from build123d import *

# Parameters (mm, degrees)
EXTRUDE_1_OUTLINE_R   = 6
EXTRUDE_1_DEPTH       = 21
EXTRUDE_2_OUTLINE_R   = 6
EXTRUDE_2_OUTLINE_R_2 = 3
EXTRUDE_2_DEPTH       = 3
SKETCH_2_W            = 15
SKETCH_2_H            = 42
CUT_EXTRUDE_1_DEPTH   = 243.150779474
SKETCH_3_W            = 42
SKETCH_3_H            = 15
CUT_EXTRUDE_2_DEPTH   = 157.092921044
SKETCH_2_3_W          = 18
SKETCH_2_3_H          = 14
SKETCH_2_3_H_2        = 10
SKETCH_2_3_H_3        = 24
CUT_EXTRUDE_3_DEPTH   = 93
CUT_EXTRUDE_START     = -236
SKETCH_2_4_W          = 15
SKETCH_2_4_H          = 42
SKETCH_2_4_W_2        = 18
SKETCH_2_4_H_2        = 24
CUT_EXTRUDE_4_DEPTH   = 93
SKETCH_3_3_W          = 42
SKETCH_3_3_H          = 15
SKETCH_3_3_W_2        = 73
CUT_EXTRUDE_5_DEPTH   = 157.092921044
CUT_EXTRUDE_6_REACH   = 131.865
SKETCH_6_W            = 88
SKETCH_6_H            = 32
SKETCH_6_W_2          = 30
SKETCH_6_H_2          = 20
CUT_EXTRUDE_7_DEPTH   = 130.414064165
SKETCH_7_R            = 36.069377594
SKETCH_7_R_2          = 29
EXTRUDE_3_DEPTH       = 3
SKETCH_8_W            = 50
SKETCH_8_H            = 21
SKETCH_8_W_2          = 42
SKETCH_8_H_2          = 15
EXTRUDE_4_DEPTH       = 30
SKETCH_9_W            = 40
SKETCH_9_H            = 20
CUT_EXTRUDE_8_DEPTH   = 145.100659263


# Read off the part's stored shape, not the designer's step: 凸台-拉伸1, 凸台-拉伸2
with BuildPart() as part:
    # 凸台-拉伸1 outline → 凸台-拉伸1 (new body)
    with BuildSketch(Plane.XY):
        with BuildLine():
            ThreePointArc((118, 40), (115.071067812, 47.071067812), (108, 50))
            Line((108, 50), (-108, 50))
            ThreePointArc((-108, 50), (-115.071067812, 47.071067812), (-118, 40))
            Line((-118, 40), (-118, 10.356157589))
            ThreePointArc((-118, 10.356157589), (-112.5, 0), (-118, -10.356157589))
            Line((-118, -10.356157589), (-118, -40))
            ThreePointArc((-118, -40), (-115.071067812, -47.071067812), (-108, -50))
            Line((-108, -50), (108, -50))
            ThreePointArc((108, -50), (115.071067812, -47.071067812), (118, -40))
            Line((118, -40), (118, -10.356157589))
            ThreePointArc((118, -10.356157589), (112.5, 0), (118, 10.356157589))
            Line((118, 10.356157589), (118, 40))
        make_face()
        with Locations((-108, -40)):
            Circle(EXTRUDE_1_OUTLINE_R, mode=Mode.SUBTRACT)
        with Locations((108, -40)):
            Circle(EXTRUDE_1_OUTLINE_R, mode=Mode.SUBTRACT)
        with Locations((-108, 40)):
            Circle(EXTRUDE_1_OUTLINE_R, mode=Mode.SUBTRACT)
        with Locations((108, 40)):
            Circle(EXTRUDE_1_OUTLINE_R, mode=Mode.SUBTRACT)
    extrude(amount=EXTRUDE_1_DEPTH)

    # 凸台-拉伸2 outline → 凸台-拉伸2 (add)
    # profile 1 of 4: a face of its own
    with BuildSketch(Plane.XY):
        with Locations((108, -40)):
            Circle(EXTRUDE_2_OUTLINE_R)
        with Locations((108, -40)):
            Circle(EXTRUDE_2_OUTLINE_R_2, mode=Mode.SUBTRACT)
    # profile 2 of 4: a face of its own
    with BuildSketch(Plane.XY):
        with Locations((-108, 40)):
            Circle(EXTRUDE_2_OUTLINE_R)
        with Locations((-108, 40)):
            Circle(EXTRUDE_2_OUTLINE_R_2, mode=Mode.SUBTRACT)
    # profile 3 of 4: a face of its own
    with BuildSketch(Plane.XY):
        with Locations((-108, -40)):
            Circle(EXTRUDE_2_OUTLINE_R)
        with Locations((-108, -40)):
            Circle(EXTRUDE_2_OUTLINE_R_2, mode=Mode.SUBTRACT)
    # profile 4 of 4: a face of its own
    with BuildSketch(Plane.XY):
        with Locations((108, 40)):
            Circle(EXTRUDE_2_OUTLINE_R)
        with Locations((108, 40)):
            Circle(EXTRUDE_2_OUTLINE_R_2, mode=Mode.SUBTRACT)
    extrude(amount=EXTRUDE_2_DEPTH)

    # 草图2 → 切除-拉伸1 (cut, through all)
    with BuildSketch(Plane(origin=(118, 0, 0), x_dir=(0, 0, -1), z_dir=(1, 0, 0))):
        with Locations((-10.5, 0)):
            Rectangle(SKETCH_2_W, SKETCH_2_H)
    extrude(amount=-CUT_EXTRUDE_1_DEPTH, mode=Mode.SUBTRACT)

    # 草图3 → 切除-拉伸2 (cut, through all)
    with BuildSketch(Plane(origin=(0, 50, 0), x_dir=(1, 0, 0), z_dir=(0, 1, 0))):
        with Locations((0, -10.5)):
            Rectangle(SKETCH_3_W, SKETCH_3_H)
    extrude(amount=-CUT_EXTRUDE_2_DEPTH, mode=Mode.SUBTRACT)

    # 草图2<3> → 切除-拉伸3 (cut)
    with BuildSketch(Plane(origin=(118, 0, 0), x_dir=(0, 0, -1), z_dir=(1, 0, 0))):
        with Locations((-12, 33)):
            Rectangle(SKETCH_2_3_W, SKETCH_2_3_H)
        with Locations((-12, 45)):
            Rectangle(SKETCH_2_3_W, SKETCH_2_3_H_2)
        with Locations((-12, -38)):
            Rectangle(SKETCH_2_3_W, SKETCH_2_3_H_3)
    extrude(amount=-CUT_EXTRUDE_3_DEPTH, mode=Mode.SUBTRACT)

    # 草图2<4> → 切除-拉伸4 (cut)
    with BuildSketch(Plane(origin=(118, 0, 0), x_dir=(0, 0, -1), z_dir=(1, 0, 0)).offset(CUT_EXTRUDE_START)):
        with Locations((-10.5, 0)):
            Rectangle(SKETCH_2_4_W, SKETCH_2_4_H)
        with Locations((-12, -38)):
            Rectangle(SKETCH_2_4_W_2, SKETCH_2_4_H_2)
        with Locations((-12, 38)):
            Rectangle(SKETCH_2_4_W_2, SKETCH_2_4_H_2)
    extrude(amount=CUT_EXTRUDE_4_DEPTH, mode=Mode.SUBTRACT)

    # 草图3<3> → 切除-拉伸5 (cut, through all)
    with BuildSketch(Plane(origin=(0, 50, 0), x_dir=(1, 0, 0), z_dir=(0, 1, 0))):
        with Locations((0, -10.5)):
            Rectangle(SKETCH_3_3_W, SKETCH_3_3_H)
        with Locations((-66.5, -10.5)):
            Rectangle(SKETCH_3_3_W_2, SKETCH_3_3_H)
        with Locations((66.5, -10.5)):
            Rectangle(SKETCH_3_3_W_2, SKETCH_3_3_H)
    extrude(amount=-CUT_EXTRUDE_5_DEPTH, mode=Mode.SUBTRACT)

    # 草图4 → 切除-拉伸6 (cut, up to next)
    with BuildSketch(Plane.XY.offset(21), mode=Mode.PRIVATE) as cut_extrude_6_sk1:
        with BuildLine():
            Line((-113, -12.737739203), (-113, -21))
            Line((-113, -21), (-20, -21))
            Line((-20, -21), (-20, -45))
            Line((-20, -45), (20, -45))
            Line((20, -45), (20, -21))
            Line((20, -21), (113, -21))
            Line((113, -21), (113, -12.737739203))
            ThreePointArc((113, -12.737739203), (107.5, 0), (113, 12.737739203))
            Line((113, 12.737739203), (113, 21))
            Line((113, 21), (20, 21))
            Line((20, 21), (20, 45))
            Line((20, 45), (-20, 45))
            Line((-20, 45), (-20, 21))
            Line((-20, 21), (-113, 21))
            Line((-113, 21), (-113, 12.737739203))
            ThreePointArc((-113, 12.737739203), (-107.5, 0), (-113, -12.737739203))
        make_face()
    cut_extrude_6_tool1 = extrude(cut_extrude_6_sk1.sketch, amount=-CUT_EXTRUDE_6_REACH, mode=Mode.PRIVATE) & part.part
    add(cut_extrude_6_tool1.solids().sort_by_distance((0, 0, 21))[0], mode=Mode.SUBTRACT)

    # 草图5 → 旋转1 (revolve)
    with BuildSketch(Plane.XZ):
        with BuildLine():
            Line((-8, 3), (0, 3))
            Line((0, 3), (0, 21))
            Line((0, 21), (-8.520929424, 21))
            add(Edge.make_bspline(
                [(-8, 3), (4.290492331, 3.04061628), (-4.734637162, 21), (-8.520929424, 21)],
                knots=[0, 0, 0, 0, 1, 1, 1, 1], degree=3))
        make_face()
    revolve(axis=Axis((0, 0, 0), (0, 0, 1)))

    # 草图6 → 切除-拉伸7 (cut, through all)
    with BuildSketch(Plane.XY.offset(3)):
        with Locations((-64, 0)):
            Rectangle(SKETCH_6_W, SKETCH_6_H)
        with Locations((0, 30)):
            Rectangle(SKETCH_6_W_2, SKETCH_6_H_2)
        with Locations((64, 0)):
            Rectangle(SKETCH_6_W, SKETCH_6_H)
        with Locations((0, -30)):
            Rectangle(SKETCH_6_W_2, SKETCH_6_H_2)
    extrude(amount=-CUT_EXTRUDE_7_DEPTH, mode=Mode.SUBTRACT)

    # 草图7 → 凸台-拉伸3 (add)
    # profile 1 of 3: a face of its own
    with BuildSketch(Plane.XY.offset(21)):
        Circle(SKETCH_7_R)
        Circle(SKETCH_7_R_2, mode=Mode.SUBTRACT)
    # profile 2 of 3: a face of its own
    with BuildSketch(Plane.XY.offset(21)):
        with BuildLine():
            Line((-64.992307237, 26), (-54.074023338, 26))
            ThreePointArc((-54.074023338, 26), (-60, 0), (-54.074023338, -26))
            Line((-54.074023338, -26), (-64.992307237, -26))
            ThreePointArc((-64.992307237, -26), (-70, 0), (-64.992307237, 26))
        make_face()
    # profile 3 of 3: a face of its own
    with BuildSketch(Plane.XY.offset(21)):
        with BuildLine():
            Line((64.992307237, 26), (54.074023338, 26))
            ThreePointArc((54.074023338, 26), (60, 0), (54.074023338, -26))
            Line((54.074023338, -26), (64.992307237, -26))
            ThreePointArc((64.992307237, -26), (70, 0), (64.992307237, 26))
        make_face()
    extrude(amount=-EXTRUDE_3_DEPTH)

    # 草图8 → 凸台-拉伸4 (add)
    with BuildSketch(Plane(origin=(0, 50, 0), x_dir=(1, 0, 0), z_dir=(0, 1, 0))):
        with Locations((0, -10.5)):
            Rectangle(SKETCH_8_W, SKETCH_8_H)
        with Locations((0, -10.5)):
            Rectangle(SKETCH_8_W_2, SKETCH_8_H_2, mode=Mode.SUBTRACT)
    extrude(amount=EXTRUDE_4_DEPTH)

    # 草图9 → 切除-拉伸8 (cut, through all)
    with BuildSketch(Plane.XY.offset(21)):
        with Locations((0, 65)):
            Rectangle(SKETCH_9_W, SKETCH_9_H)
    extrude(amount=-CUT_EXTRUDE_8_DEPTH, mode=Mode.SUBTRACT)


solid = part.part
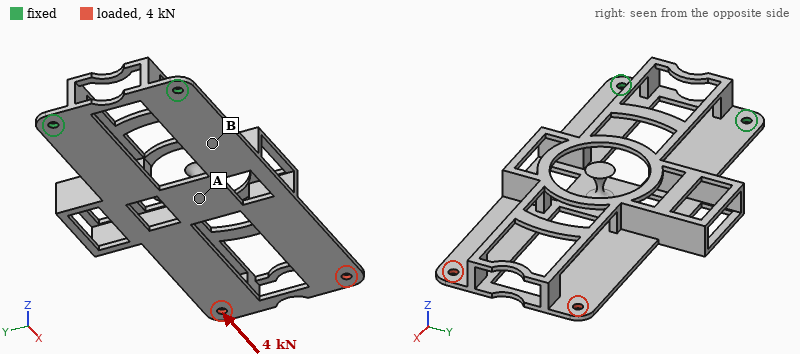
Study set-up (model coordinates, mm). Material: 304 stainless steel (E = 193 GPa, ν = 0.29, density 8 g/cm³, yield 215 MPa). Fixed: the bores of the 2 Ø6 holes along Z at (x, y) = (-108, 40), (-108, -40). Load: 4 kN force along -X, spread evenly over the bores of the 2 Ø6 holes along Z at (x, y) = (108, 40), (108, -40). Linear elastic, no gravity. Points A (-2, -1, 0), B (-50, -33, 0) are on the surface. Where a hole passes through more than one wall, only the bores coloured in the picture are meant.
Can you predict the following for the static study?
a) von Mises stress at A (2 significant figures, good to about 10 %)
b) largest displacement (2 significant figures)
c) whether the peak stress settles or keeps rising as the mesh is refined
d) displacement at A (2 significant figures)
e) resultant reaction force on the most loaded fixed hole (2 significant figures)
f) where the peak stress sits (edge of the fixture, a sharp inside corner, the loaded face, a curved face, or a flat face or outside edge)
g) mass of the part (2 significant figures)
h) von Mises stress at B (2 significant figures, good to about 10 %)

10 MPa
0.14 mm
keeps rising
0.028 mm
2.0 kN
edge of the fixture
700 g
20 MPa
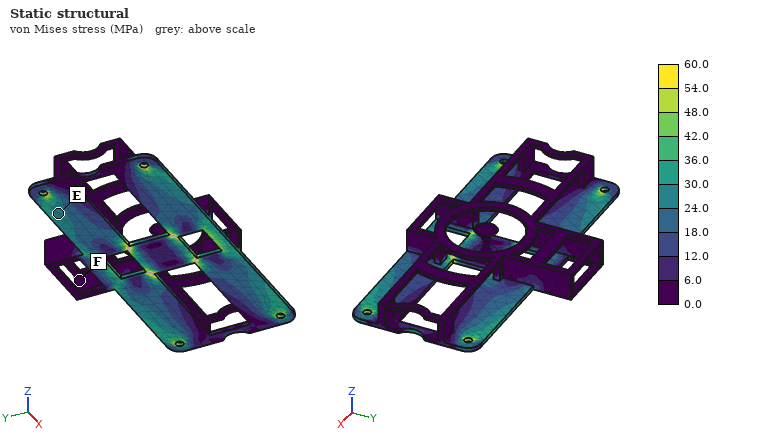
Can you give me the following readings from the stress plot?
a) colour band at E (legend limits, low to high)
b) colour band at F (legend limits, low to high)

24.0 to 30.0 MPa
0.0 to 6.0 MPa
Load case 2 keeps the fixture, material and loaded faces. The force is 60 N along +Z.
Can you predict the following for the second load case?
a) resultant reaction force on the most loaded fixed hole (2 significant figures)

37 N
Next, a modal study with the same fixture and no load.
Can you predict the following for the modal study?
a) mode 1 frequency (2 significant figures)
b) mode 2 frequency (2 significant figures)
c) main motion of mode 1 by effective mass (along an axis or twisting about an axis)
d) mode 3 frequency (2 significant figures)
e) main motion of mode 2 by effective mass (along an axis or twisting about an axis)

81 Hz
220 Hz
along Z
410 Hz
twisting about X
